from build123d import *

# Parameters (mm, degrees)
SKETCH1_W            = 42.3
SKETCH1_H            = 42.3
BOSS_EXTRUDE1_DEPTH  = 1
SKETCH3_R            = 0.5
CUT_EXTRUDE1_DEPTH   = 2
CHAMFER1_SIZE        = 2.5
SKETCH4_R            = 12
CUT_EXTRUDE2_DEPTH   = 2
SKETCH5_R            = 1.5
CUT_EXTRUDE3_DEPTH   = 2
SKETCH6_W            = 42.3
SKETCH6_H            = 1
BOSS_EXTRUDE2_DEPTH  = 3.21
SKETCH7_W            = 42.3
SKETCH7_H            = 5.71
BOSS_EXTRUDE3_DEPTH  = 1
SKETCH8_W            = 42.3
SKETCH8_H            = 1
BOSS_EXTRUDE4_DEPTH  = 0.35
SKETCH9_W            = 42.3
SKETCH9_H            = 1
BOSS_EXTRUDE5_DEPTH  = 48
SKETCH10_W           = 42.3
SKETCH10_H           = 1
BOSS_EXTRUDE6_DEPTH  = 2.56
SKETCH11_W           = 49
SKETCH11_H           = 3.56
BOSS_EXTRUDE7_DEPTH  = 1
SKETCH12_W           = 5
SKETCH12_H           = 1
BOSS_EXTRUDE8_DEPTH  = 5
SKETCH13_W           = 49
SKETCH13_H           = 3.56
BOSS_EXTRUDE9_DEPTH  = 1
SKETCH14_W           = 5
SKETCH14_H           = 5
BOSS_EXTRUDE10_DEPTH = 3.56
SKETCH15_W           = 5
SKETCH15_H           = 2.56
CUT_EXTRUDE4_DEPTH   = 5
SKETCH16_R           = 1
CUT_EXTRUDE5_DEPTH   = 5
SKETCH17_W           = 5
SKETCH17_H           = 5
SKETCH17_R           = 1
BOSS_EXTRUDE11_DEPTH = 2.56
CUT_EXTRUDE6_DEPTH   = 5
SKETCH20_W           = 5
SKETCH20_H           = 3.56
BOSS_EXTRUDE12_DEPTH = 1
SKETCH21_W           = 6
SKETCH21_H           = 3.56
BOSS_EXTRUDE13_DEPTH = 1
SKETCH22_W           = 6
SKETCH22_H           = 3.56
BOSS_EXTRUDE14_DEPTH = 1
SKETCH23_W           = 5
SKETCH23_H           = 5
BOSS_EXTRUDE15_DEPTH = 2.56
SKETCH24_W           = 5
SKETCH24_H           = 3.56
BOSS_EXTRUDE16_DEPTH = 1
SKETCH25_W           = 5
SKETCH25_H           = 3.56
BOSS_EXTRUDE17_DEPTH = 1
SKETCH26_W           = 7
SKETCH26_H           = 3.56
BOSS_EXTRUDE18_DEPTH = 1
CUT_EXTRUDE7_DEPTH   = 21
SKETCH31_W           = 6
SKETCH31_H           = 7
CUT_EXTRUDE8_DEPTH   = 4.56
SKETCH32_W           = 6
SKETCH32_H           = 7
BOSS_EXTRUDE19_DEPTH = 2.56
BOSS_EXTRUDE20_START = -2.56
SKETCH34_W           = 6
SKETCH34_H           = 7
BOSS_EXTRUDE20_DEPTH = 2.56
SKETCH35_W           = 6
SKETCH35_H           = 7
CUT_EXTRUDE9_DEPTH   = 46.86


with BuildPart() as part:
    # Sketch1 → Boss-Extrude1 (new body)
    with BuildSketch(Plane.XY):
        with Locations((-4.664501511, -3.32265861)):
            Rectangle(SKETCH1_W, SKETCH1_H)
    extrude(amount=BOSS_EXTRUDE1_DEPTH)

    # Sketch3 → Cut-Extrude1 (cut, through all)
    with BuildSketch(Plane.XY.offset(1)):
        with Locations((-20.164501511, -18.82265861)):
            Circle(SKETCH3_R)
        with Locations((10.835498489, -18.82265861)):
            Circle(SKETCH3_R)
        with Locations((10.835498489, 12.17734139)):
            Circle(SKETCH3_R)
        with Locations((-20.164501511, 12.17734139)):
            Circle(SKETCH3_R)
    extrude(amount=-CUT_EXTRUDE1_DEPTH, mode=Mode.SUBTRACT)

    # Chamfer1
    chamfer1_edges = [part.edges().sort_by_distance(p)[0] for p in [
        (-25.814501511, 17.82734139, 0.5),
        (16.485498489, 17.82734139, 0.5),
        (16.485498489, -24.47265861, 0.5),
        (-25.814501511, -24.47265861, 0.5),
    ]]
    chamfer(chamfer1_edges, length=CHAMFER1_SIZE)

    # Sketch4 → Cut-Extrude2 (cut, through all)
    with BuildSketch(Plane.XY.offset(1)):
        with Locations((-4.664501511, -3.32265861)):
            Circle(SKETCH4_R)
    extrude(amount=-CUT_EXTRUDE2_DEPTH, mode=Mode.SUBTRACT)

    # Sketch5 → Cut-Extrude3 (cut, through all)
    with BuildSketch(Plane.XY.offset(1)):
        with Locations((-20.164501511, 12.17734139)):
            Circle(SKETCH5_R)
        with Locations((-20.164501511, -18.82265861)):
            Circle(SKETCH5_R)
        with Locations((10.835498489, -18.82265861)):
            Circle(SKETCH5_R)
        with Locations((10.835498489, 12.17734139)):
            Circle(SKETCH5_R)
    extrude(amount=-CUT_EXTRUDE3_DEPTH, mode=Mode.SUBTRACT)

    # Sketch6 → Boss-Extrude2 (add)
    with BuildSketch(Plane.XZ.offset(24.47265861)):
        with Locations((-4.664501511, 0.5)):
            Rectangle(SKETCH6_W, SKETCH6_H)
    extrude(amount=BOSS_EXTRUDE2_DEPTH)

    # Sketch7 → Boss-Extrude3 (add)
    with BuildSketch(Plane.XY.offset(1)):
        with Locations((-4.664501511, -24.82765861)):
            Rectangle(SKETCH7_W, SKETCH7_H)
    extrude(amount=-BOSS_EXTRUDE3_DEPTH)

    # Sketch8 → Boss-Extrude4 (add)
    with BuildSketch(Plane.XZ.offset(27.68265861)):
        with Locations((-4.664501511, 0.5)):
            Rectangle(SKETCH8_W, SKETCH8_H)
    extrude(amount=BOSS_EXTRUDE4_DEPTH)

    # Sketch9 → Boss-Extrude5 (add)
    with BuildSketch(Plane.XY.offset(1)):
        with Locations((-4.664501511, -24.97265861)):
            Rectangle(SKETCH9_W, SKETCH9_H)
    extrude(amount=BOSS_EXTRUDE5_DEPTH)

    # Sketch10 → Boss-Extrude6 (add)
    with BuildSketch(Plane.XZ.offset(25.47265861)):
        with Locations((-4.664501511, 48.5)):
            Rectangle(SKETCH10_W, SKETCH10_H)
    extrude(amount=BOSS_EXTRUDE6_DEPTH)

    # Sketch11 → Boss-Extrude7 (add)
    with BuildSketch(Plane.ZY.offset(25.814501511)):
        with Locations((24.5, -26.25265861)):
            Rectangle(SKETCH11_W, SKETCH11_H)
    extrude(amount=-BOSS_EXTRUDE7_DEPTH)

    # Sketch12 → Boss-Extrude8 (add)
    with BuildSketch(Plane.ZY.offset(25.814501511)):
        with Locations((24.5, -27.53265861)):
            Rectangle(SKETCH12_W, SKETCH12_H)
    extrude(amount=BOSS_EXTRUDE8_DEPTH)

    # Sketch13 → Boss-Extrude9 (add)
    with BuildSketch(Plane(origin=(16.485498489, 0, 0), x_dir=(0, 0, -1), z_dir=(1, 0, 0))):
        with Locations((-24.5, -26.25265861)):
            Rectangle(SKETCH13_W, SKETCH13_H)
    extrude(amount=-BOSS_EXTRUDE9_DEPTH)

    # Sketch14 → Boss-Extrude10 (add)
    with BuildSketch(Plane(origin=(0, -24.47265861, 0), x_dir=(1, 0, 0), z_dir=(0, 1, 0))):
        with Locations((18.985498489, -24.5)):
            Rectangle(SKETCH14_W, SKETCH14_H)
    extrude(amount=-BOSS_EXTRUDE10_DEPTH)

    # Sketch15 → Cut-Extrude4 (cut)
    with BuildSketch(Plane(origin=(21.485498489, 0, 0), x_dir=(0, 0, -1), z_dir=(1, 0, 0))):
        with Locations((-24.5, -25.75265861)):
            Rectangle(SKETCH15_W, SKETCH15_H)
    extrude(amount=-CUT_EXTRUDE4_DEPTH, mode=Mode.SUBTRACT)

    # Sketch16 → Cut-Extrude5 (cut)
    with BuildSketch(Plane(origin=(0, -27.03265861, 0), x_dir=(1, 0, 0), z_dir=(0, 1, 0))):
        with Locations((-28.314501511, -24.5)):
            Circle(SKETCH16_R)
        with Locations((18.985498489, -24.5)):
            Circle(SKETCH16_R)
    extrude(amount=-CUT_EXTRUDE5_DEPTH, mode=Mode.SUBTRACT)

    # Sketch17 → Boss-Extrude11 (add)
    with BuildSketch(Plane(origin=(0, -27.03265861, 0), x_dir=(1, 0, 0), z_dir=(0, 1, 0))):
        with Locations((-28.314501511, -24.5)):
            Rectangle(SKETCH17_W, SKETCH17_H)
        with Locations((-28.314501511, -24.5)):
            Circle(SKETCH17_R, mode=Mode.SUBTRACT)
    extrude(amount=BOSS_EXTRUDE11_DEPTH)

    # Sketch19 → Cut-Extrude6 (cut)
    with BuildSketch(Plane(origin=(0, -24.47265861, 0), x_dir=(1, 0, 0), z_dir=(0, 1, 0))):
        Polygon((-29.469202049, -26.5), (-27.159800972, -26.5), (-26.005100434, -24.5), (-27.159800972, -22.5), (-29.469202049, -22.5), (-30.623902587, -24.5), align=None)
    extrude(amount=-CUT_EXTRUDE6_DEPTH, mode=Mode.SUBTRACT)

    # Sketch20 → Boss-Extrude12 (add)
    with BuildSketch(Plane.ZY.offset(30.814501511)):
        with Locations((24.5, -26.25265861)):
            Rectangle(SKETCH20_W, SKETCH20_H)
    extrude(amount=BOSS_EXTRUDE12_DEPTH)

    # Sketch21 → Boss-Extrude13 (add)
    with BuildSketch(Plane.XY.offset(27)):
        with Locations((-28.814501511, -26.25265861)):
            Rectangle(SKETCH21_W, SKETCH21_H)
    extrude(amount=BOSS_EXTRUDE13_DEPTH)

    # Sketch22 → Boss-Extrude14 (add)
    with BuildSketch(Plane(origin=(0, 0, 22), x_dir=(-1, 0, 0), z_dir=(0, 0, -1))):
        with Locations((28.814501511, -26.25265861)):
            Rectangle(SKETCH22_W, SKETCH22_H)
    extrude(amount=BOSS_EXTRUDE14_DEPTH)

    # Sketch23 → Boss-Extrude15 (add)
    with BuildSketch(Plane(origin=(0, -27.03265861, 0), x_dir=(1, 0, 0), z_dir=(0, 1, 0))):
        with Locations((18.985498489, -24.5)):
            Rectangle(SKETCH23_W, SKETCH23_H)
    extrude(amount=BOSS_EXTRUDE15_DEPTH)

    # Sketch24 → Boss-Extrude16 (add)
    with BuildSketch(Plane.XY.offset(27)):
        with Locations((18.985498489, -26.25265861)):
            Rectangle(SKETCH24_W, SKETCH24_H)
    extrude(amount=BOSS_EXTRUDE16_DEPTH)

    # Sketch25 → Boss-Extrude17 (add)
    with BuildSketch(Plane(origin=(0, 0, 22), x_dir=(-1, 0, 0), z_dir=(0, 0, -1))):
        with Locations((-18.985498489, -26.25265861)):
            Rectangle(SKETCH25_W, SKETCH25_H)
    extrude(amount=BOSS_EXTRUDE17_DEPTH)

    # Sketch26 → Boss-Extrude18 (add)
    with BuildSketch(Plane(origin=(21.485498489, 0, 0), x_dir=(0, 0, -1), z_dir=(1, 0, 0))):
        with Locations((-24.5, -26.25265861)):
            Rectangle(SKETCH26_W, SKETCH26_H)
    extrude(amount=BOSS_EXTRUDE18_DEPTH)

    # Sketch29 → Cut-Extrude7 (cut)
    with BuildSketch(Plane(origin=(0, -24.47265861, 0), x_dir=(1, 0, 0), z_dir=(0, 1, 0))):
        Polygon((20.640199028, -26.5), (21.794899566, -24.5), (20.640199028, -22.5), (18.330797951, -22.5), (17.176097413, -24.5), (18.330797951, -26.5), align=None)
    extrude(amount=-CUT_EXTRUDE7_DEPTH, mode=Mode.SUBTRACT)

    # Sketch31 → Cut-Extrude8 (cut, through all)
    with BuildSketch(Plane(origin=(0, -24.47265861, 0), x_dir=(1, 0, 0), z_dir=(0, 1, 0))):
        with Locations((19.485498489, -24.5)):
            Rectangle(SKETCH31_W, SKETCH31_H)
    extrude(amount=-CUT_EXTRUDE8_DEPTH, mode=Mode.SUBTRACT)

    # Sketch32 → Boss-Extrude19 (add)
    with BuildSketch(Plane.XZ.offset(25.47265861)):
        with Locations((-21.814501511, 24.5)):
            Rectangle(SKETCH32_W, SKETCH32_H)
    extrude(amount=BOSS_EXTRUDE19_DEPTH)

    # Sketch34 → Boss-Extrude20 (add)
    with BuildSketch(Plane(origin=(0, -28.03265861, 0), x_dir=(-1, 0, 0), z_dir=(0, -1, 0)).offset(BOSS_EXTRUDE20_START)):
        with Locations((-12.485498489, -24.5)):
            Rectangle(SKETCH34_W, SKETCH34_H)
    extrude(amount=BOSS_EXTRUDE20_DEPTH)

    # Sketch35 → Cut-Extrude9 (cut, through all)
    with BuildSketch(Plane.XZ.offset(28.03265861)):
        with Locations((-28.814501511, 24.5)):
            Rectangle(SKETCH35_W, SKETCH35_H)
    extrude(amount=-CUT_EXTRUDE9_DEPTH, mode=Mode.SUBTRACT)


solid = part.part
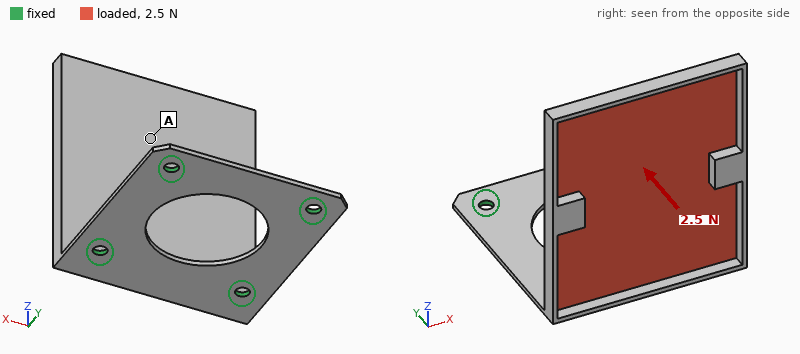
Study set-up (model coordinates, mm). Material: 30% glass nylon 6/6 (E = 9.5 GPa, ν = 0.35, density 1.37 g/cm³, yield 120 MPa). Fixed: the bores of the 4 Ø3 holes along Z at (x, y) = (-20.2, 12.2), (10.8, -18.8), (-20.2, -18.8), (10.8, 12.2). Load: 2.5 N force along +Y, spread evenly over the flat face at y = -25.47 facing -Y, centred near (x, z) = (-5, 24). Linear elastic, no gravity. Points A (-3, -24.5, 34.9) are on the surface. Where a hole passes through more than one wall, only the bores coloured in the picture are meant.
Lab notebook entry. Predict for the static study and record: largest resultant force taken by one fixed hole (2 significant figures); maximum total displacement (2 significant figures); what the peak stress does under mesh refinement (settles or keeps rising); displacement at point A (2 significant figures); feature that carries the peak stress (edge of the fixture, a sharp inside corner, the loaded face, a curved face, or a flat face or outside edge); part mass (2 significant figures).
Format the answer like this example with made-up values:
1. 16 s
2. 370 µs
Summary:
1. 1.8 N
2. 0.85 mm
3. keeps rising
4. 0.59 mm
5. edge of the fixture
6. 5.5 g
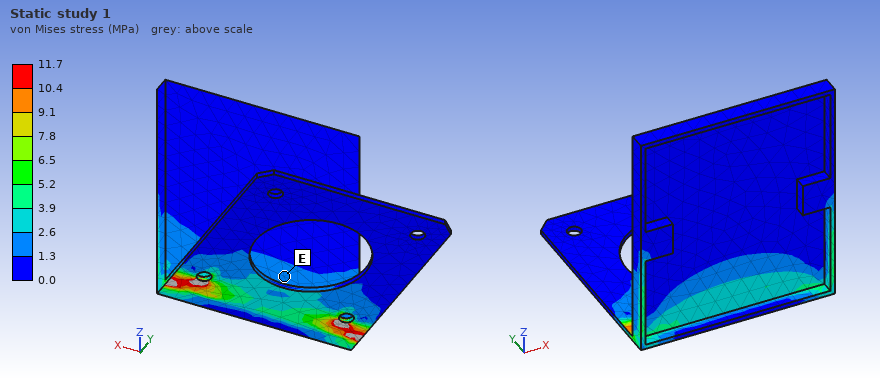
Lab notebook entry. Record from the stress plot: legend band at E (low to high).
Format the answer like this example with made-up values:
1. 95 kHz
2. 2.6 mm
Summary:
1. 1.3 to 2.6 MPa
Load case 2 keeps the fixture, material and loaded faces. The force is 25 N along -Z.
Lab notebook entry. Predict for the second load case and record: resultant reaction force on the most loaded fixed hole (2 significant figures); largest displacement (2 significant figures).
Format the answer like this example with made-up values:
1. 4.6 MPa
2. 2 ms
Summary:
1. 13 N
2. 0.89 mm
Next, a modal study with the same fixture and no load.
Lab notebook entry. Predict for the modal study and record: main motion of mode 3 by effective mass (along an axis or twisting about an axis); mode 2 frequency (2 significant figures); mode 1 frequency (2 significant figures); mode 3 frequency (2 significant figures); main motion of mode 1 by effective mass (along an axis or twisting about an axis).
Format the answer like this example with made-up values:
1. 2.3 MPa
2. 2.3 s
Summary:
1. along X
2. 460 Hz
3. 170 Hz
4. 1100 Hz
5. along Y
